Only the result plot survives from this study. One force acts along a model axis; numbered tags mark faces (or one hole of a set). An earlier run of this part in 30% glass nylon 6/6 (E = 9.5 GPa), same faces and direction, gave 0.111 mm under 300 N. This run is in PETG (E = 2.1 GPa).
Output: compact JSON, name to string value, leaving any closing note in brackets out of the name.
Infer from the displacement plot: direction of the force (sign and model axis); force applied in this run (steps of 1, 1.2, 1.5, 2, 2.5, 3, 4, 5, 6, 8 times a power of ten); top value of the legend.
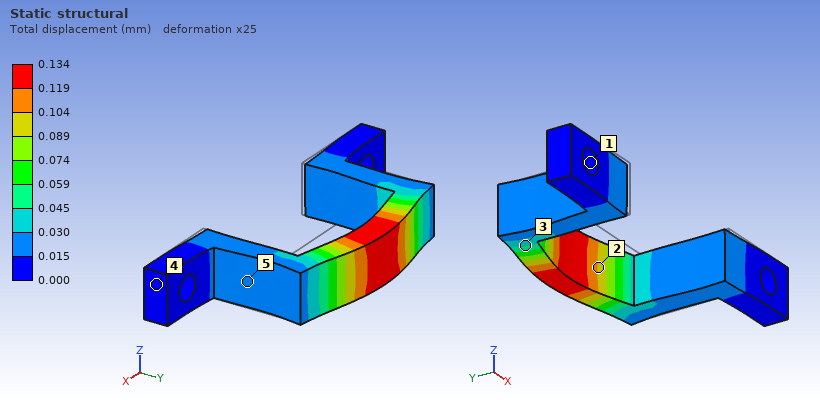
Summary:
{"direction of the force": "+Y", "force applied in this run": "80 N", "top value of the legend": "0.134 mm"}
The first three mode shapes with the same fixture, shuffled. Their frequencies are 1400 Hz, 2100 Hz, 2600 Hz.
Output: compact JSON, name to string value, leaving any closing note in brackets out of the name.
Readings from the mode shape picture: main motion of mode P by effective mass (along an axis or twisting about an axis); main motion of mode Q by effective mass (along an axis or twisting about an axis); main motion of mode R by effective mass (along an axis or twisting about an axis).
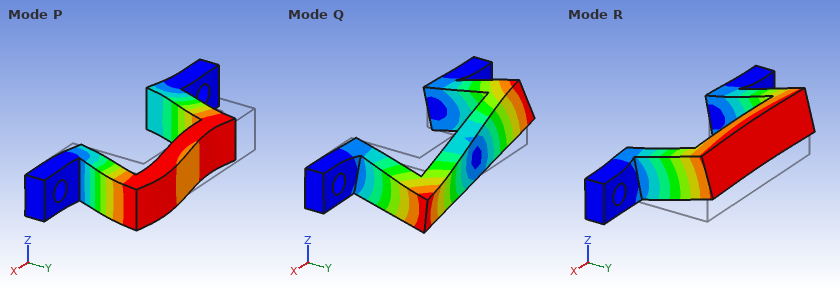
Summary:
{"main motion of mode P by effective mass": "along X", "main motion of mode Q by effective mass": "twisting about Y", "main motion of mode R by effective mass": "along Z"}
